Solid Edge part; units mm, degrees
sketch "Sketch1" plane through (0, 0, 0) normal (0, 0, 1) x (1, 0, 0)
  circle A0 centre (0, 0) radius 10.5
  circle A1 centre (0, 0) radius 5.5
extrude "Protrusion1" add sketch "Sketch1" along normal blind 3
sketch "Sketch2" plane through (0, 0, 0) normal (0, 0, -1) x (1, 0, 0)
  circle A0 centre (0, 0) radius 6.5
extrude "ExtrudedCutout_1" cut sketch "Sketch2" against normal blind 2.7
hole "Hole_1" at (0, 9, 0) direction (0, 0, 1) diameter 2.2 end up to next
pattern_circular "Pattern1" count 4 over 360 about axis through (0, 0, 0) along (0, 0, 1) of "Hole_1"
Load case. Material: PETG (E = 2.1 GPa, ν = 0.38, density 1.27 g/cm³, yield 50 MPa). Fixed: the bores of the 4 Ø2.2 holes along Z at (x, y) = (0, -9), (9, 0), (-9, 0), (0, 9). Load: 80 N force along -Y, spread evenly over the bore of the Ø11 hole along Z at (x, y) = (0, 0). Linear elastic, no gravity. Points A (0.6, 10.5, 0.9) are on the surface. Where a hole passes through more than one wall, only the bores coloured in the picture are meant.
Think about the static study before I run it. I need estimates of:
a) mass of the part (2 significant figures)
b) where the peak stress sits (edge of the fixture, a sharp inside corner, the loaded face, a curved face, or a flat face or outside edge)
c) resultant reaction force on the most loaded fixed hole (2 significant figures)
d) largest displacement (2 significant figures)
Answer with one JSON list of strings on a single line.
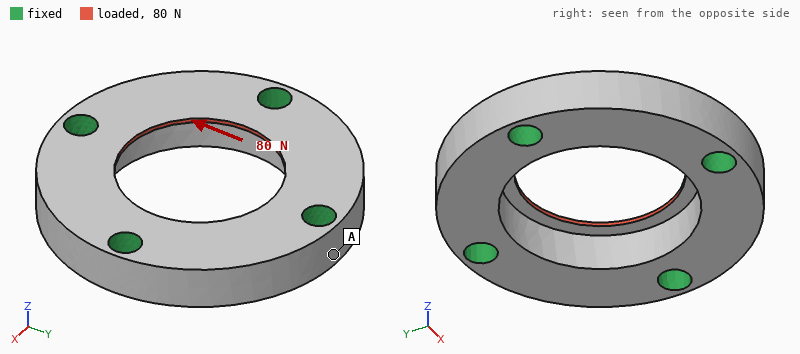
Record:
["0.77 g", "a sharp inside corner", "22 N", "18 µm"]
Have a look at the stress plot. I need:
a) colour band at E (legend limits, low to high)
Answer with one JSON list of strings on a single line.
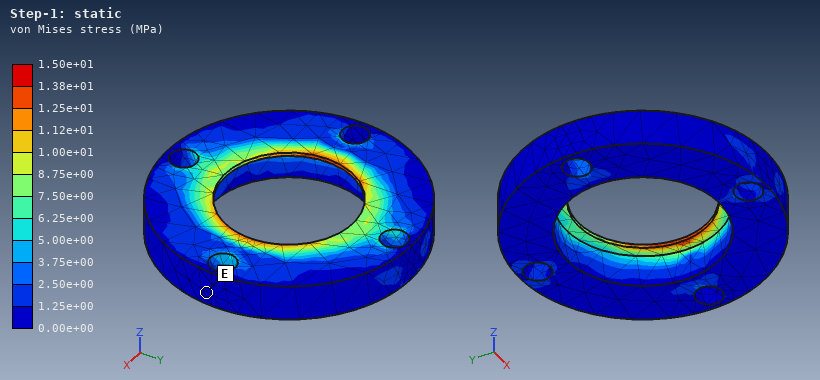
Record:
["0.00e+00 to 1.25e+00 MPa"]
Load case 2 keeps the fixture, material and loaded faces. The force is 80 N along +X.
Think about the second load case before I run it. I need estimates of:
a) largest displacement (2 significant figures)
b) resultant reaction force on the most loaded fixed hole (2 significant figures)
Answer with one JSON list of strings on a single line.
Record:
["17 µm", "22 N"]
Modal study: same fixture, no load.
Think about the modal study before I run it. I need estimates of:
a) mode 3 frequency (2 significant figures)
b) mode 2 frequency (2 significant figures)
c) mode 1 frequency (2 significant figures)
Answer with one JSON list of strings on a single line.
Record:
["18 kHz", "18 kHz", "18 kHz"]
